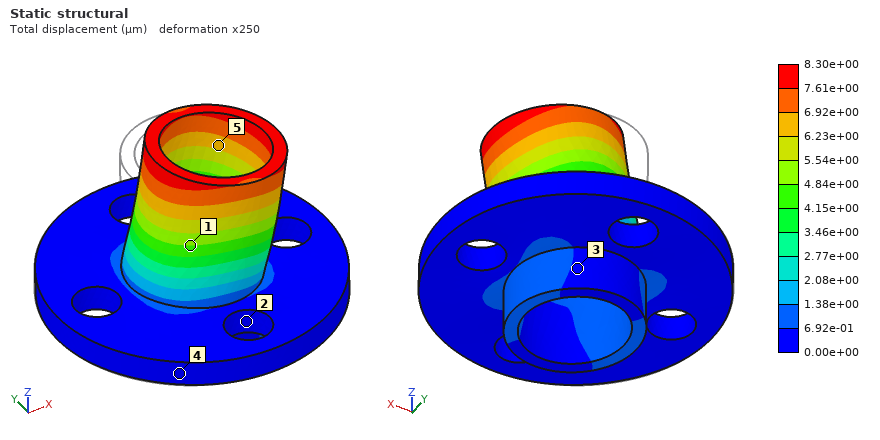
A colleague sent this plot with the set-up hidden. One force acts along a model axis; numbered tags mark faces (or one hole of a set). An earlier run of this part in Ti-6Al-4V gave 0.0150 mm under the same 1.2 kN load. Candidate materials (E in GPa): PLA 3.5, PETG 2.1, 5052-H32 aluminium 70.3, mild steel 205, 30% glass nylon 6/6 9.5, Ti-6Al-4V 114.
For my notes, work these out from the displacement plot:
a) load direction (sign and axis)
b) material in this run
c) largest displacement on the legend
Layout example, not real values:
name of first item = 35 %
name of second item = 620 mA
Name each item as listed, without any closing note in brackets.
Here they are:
load direction = +X
material in this run = mild steel
largest displacement on the legend = 8.30e+00 µm
